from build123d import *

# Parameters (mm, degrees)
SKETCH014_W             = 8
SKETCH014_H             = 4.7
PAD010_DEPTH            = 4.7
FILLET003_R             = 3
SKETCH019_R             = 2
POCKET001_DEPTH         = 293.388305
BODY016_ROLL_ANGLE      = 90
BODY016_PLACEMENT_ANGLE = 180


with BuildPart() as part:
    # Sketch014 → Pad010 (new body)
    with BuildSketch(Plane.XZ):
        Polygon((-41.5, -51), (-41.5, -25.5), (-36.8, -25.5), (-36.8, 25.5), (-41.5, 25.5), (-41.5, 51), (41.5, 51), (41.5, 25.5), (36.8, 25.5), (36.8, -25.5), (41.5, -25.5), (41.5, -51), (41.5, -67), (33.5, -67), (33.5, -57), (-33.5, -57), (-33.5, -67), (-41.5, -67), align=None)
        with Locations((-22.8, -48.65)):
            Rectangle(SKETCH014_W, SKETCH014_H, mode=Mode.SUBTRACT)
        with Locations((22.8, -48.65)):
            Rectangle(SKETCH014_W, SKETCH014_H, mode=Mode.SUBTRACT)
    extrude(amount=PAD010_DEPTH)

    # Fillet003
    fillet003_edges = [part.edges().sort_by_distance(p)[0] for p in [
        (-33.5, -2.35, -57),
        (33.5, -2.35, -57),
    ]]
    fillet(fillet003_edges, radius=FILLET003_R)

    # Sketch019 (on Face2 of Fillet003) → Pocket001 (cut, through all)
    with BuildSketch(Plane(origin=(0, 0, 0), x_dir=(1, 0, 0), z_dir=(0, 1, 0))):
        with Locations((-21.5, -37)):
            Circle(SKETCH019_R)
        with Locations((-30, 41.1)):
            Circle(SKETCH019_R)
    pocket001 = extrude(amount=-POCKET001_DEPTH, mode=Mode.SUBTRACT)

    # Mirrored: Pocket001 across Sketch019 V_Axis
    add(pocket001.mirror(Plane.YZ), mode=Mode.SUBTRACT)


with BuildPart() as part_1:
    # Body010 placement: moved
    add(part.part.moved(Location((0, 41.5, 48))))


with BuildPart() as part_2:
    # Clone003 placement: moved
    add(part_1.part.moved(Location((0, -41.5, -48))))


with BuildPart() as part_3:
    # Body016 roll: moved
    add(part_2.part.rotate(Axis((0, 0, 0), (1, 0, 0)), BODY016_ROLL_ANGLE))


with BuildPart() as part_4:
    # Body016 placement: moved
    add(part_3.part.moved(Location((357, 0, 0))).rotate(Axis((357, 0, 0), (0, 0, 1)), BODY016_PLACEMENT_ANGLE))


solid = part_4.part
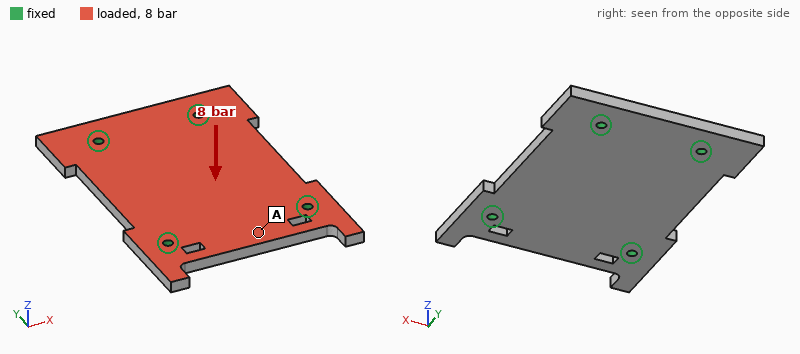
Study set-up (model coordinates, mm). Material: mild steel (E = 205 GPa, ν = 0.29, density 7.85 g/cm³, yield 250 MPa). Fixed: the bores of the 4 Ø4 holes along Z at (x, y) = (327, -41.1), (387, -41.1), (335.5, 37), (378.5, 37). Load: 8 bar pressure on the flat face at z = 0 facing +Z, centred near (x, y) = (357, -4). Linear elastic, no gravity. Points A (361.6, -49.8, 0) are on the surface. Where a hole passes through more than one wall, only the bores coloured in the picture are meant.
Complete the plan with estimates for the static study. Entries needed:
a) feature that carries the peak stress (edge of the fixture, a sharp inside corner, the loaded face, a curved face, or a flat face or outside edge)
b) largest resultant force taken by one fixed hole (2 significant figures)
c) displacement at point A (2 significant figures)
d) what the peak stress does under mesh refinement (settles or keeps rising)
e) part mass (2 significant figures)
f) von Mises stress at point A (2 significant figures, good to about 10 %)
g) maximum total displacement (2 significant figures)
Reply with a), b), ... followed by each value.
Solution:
a) edge of the fixture
b) 1.7 kN
c) 19 µm
d) keeps rising
e) 310 g
f) 38 MPa
g) 64 µm
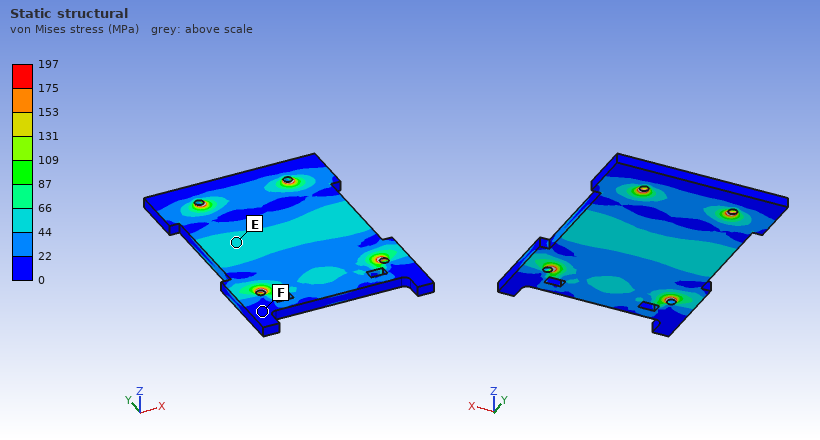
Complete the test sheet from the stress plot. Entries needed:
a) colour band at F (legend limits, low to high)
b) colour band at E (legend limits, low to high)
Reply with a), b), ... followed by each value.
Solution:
a) 0 to 22 MPa
b) 44 to 66 MPa
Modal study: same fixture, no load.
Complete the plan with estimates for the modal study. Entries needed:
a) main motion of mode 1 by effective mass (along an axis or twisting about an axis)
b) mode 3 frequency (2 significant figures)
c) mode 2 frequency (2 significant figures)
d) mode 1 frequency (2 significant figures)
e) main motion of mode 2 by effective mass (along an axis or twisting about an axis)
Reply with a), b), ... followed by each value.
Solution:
a) along Z
b) 5600 Hz
c) 4600 Hz
d) 3300 Hz
e) twisting about Y
